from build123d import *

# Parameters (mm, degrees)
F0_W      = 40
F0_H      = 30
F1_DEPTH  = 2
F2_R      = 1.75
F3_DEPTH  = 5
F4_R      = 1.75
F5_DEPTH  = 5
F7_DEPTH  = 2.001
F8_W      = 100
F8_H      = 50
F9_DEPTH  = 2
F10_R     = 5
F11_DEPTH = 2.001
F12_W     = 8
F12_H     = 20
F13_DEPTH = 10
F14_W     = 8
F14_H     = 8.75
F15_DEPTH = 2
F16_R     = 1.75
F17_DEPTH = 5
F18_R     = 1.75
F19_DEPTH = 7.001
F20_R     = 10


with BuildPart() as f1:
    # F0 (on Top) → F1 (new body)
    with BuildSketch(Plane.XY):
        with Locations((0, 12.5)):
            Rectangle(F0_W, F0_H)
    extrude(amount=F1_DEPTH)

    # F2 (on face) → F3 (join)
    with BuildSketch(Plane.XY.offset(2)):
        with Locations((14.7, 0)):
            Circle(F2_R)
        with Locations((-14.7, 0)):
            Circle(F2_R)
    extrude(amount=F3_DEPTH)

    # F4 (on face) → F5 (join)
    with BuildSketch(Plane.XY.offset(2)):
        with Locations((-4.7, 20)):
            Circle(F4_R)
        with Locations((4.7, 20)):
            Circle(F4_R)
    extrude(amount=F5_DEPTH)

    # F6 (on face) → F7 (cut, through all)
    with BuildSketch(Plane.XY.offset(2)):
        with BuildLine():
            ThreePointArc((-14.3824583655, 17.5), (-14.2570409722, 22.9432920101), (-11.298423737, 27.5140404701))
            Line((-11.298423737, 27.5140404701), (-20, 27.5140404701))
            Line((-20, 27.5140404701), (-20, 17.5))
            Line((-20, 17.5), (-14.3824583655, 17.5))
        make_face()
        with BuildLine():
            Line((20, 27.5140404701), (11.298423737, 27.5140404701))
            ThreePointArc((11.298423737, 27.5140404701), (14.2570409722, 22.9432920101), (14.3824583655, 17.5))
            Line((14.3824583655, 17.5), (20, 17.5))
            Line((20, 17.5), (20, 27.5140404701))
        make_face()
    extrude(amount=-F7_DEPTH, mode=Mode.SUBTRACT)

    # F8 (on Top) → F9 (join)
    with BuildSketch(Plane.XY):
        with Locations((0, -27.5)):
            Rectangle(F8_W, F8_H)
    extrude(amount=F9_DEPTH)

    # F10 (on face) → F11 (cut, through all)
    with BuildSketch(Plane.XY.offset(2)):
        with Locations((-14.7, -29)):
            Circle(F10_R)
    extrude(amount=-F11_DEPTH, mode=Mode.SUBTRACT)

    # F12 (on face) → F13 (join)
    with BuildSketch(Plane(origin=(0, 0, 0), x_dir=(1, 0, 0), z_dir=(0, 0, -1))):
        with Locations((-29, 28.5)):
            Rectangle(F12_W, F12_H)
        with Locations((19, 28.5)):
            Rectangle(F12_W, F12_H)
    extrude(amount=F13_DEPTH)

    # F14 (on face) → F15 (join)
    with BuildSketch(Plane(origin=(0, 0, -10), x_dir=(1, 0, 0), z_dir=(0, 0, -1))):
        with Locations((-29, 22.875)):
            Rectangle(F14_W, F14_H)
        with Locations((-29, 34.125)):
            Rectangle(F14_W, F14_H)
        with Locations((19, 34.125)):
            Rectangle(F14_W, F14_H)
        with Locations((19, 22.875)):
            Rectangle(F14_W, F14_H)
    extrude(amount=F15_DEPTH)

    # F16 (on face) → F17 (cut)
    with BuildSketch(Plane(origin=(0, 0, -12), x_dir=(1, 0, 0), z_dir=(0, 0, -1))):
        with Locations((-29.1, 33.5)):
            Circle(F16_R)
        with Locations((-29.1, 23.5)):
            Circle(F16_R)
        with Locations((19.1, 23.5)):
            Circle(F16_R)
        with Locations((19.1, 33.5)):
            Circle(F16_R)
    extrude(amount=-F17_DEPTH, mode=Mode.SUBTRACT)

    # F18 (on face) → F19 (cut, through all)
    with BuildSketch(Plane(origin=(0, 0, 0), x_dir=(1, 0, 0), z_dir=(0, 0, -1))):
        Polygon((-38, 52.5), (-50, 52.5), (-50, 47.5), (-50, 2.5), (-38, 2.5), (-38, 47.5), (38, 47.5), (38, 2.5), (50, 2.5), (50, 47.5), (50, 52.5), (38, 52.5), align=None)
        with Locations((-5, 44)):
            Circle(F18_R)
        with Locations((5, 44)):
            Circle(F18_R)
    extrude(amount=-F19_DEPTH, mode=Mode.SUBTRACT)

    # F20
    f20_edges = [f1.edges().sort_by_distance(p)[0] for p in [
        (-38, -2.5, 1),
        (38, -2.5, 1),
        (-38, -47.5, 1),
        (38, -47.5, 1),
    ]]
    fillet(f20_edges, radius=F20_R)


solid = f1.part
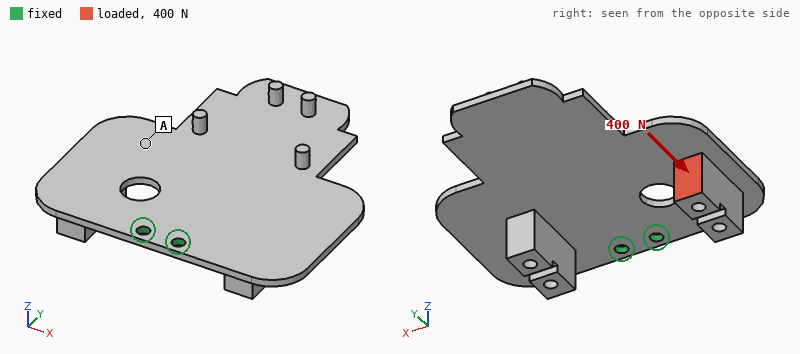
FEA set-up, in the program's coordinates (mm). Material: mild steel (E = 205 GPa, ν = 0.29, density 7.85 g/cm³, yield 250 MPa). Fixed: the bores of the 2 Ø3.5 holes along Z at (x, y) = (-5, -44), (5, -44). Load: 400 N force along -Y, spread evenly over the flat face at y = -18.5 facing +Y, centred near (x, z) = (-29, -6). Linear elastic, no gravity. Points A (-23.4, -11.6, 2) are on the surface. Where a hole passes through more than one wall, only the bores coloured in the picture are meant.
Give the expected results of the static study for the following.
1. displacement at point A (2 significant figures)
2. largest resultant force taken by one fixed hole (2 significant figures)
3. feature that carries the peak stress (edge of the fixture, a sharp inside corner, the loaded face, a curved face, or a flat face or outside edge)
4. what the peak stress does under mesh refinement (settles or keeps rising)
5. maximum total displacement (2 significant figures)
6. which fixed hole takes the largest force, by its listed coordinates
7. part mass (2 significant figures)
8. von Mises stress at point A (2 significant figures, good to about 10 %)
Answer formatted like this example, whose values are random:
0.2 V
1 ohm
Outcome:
0.23 mm
1.0 kN
edge of the fixture
keeps rising
0.42 mm
(-5, -44)
97 g
29 MPa
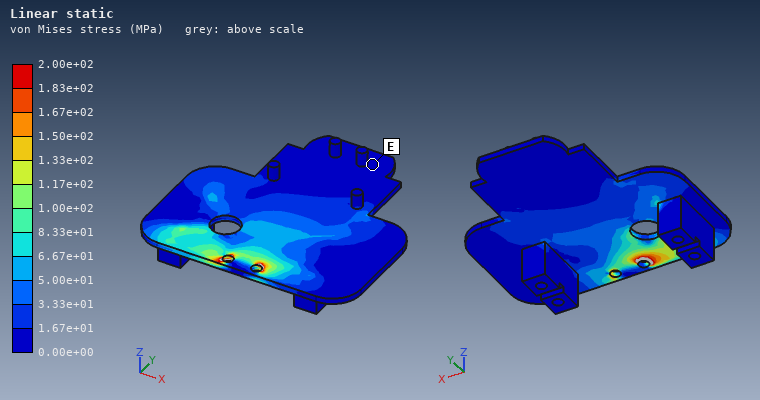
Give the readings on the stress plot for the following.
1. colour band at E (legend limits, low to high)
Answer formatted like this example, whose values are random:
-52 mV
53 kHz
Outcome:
0.00e+00 to 1.67e+01 MPa
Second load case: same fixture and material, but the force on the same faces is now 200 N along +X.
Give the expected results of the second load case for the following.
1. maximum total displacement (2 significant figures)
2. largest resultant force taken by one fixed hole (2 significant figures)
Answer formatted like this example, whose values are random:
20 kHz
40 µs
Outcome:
0.18 mm
390 N
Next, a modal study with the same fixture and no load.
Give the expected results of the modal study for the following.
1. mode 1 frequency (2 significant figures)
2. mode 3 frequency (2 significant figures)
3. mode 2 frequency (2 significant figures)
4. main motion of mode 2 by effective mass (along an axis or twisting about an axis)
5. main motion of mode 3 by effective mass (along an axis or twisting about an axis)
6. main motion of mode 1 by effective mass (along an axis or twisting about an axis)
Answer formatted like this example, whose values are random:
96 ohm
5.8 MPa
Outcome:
380 Hz
1100 Hz
620 Hz
twisting about Y
along Z
along Z
